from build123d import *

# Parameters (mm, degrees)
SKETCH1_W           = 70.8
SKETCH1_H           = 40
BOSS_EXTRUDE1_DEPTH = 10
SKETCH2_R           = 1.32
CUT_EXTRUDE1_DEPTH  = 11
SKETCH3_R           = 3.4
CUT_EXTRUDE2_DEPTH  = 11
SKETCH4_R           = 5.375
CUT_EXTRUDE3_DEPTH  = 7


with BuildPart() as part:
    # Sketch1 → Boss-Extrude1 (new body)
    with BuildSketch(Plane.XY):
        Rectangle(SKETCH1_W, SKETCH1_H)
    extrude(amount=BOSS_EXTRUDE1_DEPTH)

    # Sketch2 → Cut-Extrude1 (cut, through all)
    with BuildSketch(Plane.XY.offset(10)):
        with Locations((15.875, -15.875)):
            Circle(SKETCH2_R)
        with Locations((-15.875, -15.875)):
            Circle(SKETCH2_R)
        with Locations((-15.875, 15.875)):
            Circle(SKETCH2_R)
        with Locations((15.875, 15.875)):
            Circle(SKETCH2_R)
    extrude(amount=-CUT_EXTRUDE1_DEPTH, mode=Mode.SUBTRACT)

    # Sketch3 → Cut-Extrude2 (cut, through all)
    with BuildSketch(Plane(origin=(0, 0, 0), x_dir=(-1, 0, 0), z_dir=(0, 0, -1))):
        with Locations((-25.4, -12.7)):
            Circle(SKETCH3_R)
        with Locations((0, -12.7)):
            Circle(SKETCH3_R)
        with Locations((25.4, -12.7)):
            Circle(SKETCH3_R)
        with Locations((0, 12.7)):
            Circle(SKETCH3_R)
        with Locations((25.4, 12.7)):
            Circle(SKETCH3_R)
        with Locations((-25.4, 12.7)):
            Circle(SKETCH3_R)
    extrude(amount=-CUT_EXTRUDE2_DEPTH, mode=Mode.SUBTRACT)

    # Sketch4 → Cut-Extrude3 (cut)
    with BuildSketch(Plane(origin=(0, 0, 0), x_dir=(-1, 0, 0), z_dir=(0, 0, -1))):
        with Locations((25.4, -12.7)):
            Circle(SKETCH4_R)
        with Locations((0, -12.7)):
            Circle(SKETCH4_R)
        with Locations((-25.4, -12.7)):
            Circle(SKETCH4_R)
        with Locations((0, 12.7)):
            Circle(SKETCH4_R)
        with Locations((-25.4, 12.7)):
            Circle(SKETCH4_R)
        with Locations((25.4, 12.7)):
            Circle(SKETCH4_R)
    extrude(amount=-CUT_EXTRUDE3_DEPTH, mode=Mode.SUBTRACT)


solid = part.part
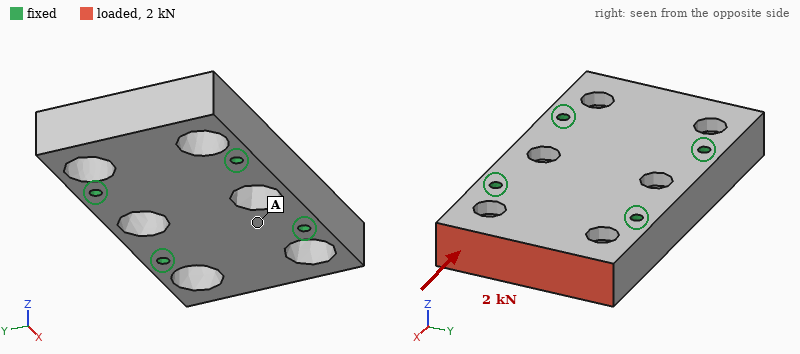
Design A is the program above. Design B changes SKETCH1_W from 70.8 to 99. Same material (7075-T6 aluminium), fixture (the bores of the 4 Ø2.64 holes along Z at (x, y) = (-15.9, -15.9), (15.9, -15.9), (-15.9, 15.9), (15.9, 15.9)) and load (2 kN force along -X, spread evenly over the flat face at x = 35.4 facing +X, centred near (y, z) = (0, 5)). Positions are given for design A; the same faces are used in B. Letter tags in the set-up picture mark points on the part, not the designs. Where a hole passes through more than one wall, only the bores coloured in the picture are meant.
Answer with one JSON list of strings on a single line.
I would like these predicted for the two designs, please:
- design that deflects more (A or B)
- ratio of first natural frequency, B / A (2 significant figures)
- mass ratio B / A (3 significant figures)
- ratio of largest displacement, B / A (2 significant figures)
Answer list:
["B", "0.39", "1.48", "1.1"]
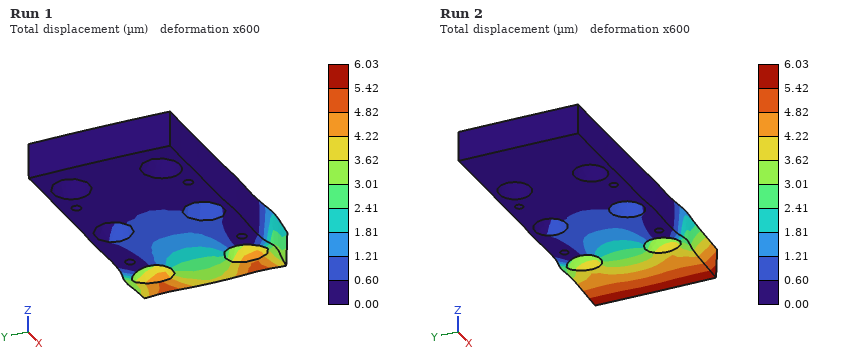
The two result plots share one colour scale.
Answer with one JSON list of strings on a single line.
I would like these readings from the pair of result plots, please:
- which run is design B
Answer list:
["Run 2"]
